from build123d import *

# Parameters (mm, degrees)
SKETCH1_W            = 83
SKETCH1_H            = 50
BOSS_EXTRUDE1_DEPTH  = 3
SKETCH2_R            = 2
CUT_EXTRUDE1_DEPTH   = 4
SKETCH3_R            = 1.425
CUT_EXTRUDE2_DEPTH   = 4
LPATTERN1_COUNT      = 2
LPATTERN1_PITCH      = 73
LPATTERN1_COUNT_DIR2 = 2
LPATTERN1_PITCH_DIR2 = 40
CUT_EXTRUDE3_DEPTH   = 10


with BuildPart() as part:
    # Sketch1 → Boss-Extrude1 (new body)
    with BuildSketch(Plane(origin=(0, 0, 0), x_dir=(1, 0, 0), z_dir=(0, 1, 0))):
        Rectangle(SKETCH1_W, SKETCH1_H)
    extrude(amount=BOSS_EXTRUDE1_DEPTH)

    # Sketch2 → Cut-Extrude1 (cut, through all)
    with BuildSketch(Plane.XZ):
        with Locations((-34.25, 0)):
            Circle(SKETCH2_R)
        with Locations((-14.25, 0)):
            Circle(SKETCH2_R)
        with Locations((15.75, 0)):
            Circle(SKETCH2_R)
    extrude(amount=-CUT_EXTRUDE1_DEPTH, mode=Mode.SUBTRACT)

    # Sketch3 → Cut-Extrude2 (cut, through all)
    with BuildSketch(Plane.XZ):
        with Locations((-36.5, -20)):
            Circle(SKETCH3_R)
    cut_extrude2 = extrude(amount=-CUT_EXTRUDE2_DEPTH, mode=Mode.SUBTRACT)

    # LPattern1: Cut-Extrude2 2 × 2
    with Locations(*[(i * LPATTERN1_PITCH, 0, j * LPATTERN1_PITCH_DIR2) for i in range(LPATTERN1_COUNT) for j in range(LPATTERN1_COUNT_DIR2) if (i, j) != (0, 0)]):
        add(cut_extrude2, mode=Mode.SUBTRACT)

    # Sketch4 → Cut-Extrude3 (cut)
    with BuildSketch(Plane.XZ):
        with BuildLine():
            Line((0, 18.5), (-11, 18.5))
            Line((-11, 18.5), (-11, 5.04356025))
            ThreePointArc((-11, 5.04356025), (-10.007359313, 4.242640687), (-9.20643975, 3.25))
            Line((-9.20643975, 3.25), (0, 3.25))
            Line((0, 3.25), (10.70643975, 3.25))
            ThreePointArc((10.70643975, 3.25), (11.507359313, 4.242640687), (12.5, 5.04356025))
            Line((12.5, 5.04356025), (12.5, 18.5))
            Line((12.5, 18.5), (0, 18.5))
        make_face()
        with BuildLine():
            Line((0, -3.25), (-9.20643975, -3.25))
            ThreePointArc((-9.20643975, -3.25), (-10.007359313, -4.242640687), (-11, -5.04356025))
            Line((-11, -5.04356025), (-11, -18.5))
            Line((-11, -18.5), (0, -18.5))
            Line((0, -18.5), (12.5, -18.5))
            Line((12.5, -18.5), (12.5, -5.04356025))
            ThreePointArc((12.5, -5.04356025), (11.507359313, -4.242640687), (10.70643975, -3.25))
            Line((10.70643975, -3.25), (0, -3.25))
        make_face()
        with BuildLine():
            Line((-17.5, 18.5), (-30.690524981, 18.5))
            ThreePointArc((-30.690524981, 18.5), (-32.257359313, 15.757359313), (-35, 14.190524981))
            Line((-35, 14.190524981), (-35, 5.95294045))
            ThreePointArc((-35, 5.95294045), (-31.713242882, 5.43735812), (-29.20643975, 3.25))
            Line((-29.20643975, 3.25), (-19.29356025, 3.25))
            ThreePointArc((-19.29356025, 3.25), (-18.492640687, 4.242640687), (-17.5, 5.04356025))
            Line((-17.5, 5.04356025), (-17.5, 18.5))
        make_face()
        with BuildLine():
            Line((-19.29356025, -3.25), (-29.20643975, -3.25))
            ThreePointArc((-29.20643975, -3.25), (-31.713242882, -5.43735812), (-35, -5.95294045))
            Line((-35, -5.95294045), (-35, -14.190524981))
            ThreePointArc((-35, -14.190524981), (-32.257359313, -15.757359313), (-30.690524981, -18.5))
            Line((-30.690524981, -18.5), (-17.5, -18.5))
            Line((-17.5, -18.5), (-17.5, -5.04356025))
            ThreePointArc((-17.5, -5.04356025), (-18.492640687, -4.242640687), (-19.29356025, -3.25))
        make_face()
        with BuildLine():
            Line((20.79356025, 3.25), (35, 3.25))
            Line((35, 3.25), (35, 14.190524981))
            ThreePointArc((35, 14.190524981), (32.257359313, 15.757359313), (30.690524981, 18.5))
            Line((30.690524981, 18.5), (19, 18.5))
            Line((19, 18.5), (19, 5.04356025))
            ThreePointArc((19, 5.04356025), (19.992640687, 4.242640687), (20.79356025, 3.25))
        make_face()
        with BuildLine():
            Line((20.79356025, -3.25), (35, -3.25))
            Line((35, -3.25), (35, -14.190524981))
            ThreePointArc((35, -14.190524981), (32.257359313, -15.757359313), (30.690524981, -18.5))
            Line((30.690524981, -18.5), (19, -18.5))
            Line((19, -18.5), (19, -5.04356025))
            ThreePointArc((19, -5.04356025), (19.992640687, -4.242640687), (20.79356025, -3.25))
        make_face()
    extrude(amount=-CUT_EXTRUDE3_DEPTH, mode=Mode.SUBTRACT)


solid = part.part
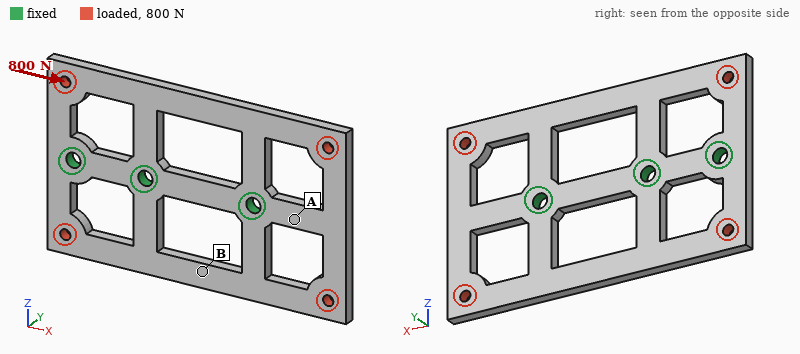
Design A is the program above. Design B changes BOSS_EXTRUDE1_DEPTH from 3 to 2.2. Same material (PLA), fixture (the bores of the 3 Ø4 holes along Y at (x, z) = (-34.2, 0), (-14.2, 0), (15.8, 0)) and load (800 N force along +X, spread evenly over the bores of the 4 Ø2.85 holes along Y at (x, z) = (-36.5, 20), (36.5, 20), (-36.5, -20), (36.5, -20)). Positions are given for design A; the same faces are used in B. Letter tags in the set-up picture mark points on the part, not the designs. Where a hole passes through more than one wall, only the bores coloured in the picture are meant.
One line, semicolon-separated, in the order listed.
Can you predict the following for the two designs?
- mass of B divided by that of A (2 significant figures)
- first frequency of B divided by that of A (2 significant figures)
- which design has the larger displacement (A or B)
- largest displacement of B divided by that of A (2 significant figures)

0.73; 0.75; B; 1.3
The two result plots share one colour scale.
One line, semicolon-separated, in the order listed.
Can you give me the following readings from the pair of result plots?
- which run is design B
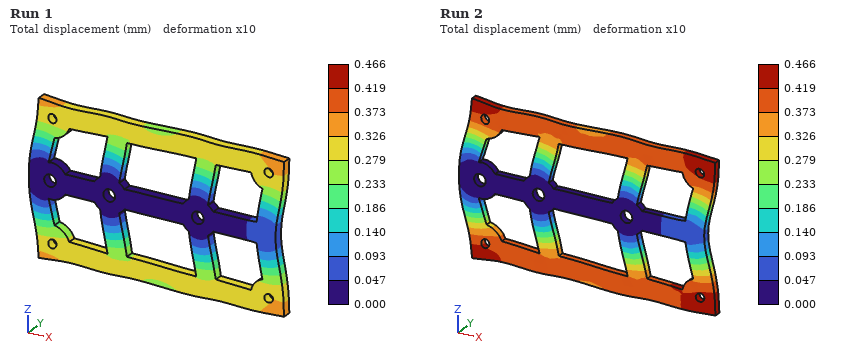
Run 2
